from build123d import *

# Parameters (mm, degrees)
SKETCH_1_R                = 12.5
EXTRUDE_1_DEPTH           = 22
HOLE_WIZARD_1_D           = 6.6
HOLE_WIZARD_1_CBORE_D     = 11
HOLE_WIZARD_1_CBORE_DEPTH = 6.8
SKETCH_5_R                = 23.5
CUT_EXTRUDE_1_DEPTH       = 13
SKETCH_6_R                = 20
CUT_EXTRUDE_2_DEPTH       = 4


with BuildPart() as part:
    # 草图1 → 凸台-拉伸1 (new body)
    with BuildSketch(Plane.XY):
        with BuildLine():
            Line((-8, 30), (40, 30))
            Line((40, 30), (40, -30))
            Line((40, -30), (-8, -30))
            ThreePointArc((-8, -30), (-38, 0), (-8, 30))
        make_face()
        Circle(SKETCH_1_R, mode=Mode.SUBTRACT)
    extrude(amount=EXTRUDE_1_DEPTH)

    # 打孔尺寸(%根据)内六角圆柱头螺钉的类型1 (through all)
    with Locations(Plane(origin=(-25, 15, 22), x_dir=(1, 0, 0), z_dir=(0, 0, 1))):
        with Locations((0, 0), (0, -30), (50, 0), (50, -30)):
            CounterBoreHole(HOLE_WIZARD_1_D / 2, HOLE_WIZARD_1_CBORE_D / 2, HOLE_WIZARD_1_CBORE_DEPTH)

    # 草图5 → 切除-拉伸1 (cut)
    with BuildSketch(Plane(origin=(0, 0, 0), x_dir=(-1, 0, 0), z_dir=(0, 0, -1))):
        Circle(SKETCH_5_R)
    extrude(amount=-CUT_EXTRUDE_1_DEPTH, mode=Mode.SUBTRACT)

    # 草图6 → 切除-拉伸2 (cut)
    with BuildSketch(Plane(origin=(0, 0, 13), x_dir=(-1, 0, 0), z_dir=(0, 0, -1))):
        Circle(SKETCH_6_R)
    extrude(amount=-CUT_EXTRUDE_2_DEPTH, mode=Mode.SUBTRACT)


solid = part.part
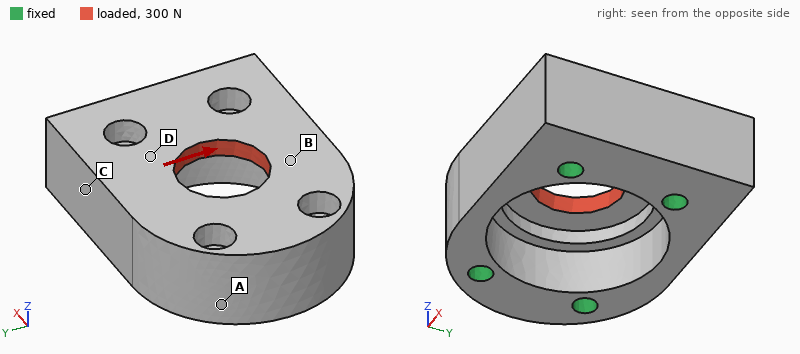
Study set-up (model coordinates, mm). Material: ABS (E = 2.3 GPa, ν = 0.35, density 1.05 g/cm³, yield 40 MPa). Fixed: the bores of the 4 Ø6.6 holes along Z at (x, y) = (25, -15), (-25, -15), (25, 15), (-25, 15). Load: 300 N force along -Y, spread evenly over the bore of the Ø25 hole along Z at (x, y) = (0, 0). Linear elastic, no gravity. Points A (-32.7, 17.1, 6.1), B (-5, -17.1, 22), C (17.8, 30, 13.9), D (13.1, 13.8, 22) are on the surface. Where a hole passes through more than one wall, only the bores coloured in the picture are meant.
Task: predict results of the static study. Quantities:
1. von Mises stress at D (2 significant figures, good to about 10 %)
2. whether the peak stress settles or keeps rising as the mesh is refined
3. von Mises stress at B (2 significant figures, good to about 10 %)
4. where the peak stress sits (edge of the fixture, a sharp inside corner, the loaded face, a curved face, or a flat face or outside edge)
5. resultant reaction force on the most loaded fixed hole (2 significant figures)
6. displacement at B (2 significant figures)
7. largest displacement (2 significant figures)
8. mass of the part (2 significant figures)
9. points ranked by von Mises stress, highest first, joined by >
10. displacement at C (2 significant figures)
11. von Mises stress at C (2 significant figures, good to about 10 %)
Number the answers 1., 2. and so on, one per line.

1. 0.93 MPa
2. keeps rising
3. 0.77 MPa
4. edge of the fixture
5. 81 N
6. 15 µm
7. 18 µm
8. 63 g
9. D > B > C > A
10. 5.8 µm
11. 0.35 MPa
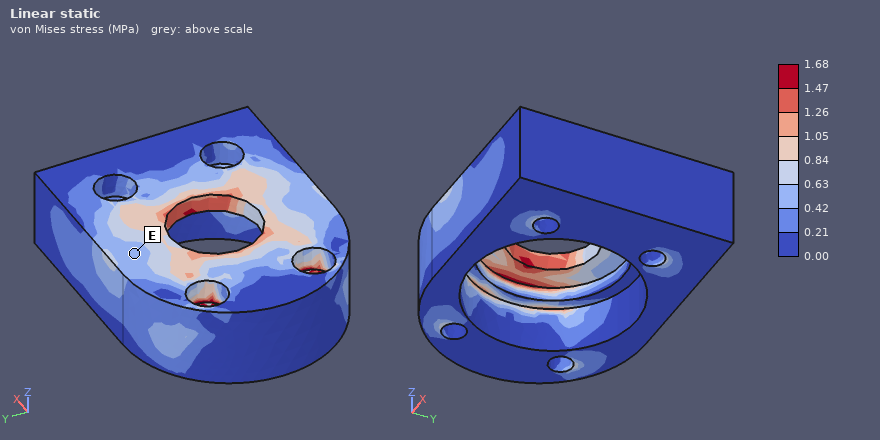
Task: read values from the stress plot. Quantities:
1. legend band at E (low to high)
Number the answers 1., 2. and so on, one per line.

1. 0.42 to 0.63 MPa
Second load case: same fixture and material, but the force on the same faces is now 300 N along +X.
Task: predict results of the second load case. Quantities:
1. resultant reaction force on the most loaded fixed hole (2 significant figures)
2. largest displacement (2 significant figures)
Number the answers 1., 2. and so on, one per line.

1. 80 N
2. 15 µm
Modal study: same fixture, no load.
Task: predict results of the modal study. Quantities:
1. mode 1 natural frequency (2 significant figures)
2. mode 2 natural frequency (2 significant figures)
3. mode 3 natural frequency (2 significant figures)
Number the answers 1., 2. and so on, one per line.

1. 5700 Hz
2. 5800 Hz
3. 6900 Hz
